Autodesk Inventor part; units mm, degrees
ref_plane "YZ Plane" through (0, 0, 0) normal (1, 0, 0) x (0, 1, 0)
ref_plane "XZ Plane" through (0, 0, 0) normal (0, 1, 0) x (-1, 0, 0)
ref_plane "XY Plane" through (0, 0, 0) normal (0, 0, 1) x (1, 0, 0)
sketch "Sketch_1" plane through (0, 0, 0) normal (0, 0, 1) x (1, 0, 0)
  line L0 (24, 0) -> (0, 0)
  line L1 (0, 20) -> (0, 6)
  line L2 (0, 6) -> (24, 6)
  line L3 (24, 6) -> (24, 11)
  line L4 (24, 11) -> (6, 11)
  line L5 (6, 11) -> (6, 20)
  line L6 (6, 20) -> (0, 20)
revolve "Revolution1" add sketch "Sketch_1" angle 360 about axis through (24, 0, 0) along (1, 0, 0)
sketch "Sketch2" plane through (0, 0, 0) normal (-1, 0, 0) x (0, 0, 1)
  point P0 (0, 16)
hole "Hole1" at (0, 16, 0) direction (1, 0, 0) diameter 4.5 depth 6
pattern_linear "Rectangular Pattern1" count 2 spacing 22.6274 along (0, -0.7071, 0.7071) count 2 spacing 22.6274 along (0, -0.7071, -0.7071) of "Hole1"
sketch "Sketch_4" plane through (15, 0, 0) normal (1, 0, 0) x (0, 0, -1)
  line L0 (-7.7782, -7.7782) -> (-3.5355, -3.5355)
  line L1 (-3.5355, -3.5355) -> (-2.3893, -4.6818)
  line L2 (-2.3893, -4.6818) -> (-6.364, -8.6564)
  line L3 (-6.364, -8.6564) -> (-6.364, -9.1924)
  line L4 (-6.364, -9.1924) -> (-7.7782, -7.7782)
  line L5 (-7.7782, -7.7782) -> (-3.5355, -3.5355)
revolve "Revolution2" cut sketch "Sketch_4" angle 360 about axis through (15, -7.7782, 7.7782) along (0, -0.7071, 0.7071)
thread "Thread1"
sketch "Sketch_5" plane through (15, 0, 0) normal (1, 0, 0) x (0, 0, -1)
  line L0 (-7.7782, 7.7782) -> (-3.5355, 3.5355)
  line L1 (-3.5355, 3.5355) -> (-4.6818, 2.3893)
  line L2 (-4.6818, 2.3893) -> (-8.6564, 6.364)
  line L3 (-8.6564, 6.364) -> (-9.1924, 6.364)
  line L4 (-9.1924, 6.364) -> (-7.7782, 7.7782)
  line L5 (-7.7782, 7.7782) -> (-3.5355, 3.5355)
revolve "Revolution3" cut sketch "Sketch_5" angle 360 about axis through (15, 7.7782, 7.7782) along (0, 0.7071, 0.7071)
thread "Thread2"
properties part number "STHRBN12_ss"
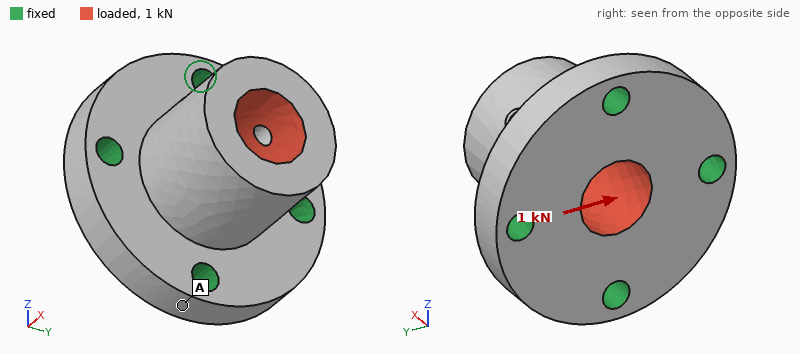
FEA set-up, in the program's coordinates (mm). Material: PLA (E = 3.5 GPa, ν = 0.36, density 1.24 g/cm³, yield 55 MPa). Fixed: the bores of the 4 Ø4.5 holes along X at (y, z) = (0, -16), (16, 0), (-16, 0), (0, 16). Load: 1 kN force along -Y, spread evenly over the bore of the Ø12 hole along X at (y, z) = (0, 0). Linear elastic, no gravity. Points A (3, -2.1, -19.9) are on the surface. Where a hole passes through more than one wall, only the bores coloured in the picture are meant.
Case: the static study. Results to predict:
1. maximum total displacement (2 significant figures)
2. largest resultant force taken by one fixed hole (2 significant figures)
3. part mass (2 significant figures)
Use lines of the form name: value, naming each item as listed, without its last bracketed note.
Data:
maximum total displacement: 0.11 mm
largest resultant force taken by one fixed hole: 440 N
part mass: 14 g
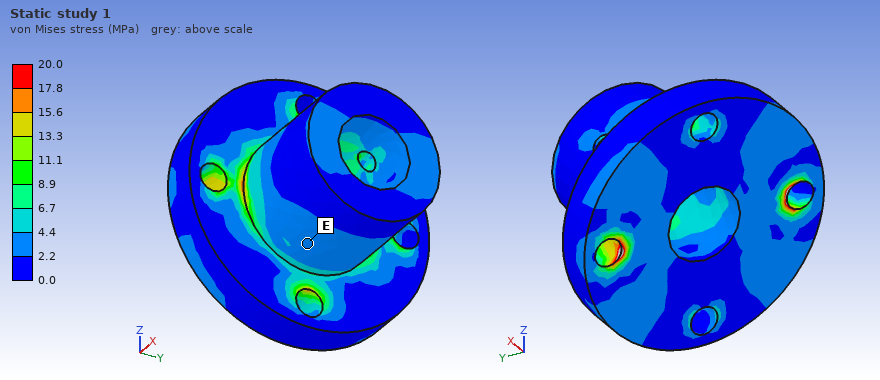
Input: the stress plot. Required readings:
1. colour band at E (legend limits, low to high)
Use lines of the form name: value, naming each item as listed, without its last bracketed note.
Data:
colour band at E: 2.2 to 4.4 MPa
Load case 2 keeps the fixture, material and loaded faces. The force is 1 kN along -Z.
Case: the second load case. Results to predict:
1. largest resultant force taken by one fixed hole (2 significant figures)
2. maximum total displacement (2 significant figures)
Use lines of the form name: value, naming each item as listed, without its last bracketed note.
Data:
largest resultant force taken by one fixed hole: 440 N
maximum total displacement: 0.11 mm
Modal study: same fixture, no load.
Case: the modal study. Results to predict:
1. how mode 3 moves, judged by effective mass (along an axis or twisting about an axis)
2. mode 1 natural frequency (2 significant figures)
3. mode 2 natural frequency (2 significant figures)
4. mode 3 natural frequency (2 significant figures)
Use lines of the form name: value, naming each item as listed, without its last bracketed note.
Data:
how mode 3 moves, judged by effective mass: along X
mode 1 natural frequency: 6400 Hz
mode 2 natural frequency: 6400 Hz
mode 3 natural frequency: 10 kHz
